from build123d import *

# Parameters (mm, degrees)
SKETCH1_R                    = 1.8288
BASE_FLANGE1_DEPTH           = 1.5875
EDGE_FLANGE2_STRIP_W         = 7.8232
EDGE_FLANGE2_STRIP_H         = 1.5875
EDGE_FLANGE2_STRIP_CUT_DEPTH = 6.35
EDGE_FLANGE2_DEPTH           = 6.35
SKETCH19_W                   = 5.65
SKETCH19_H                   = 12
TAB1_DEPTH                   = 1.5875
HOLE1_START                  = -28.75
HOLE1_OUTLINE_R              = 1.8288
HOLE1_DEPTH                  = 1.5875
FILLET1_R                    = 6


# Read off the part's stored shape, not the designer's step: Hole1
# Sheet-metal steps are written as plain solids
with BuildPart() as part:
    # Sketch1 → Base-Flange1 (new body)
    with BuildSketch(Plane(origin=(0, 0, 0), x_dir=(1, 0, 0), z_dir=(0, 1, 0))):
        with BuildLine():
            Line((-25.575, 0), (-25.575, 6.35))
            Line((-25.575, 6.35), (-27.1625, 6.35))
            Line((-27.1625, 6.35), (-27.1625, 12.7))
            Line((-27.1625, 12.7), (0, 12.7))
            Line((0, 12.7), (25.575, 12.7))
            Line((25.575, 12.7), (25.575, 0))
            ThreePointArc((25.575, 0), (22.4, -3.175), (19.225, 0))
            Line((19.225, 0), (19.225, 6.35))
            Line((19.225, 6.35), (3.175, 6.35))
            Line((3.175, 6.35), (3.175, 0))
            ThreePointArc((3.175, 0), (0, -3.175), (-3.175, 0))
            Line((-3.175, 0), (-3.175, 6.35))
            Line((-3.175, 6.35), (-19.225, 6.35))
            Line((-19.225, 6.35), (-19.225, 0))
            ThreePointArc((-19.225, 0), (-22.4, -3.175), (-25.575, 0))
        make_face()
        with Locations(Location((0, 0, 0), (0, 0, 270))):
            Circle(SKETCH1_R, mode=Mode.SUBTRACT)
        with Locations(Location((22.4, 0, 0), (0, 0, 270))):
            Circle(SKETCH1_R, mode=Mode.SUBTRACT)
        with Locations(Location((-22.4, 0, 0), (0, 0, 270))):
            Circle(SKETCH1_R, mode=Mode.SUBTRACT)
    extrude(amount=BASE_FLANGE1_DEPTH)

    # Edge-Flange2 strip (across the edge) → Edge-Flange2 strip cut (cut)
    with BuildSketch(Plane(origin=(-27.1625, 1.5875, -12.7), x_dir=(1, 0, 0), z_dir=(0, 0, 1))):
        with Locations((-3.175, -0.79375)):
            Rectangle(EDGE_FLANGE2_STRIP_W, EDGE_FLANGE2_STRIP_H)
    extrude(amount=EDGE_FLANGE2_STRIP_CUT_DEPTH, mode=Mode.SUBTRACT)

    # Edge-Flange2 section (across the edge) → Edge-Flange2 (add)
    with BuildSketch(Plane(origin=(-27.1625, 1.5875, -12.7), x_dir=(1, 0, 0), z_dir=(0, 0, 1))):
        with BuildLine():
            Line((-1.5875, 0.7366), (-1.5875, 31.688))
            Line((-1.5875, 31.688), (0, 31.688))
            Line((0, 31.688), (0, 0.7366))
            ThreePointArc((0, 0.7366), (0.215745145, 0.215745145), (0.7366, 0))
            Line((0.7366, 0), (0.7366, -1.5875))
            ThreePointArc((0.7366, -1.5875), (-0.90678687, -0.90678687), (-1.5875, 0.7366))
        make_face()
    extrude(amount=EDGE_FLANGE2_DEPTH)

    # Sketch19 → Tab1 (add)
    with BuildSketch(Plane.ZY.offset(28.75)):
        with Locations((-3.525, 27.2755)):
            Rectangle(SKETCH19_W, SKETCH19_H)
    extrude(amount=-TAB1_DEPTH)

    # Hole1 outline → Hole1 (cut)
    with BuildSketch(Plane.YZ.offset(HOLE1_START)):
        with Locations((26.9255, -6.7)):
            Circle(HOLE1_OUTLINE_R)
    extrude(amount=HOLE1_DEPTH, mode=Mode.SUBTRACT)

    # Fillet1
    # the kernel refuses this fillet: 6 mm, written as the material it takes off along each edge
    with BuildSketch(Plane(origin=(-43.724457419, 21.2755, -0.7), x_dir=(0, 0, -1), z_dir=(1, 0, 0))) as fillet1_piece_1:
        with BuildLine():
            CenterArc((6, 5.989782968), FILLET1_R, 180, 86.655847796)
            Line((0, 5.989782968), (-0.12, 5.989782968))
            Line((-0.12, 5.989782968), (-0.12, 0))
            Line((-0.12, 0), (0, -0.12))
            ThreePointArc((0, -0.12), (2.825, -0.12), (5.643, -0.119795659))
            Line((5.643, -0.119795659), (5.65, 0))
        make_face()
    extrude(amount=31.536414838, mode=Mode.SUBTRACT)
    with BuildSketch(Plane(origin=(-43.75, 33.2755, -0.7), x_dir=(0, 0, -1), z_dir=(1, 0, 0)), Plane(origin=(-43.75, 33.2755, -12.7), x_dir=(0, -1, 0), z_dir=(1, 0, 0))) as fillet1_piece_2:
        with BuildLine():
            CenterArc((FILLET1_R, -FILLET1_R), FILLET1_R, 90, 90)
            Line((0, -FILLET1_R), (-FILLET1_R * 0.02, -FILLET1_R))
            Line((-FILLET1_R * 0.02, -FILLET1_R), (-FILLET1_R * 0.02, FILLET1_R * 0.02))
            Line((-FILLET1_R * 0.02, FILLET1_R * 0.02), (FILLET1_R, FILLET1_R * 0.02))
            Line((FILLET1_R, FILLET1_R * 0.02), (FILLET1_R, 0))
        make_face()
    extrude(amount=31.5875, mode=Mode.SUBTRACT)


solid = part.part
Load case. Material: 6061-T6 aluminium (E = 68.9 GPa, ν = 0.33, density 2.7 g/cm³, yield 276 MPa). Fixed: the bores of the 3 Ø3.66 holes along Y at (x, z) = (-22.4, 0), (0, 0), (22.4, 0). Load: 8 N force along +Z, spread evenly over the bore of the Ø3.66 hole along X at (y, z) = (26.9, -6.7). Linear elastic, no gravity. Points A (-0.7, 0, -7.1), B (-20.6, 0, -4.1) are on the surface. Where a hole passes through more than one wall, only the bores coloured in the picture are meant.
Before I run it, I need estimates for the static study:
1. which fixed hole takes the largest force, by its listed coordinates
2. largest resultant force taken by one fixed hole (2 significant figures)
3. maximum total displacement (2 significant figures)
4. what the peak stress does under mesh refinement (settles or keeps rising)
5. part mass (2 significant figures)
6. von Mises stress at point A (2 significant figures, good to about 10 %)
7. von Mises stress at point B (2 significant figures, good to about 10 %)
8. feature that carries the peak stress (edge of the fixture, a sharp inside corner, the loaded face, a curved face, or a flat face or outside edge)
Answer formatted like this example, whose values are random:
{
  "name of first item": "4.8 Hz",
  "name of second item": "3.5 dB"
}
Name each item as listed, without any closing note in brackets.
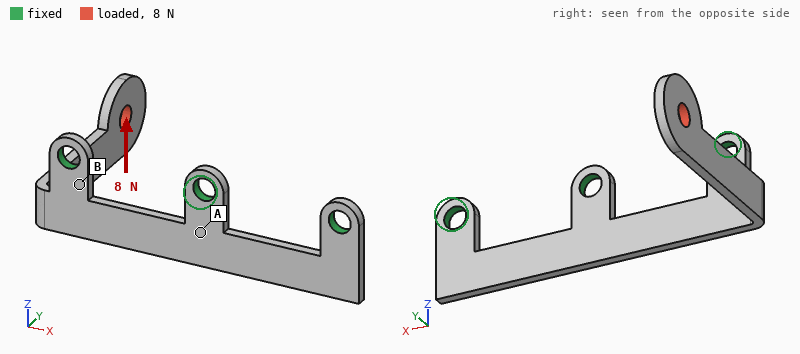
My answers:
{
  "which fixed hole takes the largest force, by its listed coordinates": "(-22.4, 0)",
  "largest resultant force taken by one fixed hole": "9.4 N",
  "maximum total displacement": "0.39 mm",
  "what the peak stress does under mesh refinement": "keeps rising",
  "part mass": "3.1 g",
  "von Mises stress at point A": "13 MPa",
  "von Mises stress at point B": "55 MPa",
  "feature that carries the peak stress": "a sharp inside corner"
}
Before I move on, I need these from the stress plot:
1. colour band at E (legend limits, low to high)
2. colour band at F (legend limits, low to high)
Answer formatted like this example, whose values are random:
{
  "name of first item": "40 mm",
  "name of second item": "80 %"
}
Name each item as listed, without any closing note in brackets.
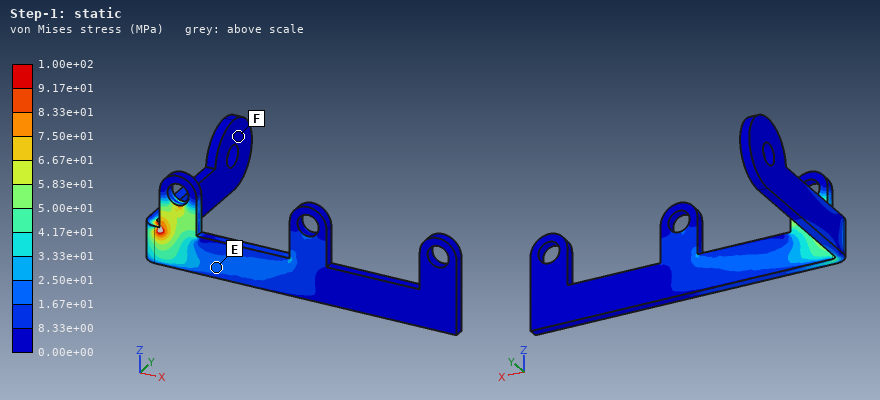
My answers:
{
  "colour band at E": "1.67e+01 to 2.50e+01 MPa",
  "colour band at F": "0.00e+00 to 8.33e+00 MPa"
}
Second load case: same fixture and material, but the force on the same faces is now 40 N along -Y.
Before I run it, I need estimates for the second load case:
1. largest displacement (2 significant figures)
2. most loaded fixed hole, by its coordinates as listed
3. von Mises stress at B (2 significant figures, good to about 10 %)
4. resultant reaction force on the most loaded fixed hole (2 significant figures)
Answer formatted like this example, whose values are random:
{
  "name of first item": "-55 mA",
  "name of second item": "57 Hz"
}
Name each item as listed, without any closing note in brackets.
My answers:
{
  "largest displacement": "0.24 mm",
  "most loaded fixed hole, by its coordinates as listed": "(-22.4, 0)",
  "von Mises stress at B": "45 MPa",
  "resultant reaction force on the most loaded fixed hole": "43 N"
}
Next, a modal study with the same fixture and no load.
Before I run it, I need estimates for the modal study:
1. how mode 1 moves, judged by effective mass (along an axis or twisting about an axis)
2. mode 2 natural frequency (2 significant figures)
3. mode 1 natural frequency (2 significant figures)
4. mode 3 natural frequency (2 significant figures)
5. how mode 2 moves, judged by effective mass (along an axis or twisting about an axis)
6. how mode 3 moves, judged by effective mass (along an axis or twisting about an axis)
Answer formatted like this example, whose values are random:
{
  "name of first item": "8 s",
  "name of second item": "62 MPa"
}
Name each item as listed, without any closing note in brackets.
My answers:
{
  "how mode 1 moves, judged by effective mass": "along X",
  "mode 2 natural frequency": "1000 Hz",
  "mode 1 natural frequency": "780 Hz",
  "mode 3 natural frequency": "4700 Hz",
  "how mode 2 moves, judged by effective mass": "along Z",
  "how mode 3 moves, judged by effective mass": "along Y"
}
